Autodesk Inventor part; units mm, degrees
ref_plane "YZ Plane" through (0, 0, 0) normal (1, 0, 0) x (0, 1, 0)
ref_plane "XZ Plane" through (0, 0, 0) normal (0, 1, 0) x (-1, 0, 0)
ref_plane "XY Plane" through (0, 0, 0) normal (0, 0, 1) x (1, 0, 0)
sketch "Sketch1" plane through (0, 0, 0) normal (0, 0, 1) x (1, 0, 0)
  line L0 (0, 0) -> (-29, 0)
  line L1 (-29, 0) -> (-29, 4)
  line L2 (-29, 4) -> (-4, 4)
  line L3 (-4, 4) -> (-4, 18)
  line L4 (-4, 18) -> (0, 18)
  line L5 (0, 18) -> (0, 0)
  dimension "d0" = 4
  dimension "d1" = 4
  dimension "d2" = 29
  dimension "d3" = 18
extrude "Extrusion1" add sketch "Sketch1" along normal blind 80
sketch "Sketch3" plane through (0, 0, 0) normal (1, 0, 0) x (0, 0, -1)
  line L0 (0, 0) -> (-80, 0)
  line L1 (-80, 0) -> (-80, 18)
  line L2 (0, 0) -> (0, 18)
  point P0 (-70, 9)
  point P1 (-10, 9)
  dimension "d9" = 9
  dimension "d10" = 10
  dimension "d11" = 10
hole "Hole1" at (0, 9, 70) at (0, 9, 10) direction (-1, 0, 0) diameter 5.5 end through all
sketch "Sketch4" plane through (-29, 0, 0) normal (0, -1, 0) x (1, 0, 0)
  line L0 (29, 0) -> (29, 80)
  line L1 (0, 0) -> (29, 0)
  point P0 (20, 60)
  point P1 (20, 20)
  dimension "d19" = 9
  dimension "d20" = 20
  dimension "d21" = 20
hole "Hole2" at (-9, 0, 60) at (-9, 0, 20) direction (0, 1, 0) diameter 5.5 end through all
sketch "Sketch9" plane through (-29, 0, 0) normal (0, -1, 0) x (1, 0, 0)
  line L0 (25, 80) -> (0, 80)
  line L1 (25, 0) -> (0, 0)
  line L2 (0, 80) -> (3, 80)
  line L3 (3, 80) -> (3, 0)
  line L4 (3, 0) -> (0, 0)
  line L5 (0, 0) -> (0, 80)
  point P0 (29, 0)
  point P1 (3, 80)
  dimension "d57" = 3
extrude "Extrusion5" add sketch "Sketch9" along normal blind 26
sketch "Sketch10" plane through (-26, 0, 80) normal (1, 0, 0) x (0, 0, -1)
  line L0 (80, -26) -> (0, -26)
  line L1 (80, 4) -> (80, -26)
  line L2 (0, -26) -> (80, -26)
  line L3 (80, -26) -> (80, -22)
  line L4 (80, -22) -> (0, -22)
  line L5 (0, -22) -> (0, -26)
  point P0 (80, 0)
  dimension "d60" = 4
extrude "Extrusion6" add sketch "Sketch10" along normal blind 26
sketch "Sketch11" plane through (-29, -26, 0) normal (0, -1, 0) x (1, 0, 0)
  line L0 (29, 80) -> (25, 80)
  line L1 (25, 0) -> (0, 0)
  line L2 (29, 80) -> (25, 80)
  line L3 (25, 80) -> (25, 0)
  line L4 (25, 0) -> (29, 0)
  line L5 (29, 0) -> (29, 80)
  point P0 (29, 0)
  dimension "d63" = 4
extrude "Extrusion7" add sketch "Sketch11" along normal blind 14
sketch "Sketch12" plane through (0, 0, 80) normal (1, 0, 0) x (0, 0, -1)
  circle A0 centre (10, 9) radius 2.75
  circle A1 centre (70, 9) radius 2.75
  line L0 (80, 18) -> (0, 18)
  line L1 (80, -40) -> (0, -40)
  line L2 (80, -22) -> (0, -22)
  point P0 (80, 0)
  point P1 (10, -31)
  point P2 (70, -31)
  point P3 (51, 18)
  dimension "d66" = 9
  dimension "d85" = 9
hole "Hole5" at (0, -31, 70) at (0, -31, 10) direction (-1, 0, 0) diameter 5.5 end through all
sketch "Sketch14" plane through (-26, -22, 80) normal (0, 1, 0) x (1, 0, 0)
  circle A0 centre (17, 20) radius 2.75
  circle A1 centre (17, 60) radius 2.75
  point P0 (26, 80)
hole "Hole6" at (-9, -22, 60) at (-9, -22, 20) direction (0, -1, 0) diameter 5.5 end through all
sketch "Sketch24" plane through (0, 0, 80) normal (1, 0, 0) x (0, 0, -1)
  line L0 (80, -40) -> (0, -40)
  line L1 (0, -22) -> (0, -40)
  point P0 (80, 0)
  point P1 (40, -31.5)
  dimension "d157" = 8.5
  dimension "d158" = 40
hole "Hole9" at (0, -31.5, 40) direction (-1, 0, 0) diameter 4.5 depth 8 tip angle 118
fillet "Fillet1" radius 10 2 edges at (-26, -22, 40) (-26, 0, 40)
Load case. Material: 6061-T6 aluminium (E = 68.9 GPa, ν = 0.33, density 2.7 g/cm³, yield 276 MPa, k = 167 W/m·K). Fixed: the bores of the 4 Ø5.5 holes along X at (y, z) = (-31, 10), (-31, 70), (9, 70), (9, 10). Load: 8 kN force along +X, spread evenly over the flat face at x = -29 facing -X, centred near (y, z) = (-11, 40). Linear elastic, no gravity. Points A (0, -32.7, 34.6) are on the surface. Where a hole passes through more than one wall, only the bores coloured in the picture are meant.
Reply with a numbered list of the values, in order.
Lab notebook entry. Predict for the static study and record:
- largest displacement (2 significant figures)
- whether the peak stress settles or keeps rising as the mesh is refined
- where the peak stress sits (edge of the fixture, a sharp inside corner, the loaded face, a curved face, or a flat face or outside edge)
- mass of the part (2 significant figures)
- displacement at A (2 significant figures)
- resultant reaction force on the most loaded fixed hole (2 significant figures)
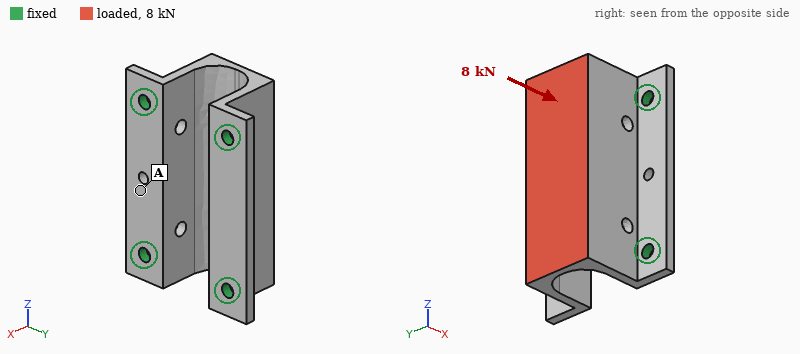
1. 38 µm
2. keeps rising
3. edge of the fixture
4. 96 g
5. 24 µm
6. 2.1 kN
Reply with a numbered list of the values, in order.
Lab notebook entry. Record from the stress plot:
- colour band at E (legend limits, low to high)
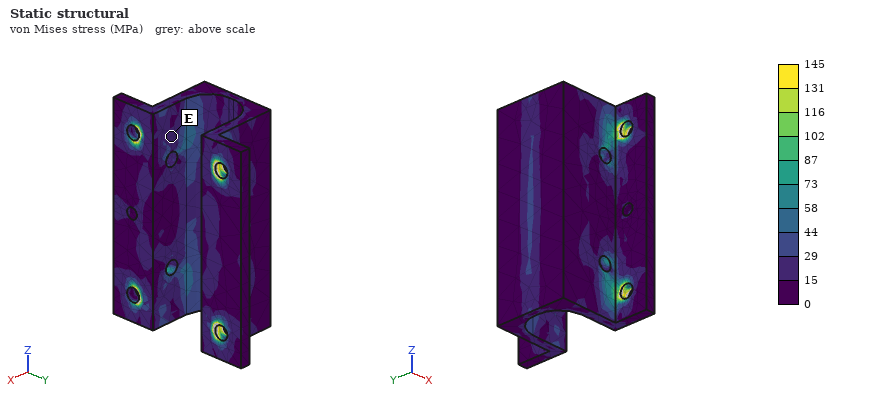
1. 15 to 29 MPa
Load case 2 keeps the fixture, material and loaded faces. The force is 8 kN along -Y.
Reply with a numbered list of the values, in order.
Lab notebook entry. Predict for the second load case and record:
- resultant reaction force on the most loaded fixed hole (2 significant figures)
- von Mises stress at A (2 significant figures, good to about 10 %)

1. 3.5 kN
2. 36 MPa
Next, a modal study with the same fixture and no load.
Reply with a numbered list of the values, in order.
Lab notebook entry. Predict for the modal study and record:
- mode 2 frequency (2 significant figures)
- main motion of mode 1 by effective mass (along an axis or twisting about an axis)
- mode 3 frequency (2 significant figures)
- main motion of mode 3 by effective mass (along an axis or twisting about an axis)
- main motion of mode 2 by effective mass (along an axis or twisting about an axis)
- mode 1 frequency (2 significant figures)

1. 7000 Hz
2. along Y
3. 9500 Hz
4. along X
5. twisting about X
6. 4800 Hz
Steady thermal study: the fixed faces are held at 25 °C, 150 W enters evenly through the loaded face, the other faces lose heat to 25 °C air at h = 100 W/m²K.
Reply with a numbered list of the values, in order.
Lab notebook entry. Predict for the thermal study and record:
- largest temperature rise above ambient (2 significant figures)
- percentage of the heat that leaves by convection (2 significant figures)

1. 47 K
2. 25 %
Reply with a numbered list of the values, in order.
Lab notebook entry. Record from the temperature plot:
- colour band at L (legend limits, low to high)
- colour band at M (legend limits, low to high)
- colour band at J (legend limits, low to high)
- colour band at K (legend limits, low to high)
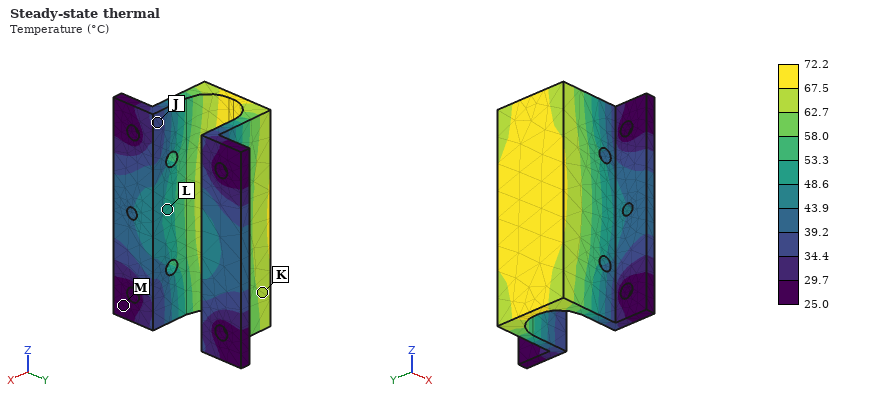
1. 48.6 to 53.3 °C
2. 25.0 to 29.7 °C
3. 34.4 to 39.2 °C
4. 62.7 to 67.5 °C
